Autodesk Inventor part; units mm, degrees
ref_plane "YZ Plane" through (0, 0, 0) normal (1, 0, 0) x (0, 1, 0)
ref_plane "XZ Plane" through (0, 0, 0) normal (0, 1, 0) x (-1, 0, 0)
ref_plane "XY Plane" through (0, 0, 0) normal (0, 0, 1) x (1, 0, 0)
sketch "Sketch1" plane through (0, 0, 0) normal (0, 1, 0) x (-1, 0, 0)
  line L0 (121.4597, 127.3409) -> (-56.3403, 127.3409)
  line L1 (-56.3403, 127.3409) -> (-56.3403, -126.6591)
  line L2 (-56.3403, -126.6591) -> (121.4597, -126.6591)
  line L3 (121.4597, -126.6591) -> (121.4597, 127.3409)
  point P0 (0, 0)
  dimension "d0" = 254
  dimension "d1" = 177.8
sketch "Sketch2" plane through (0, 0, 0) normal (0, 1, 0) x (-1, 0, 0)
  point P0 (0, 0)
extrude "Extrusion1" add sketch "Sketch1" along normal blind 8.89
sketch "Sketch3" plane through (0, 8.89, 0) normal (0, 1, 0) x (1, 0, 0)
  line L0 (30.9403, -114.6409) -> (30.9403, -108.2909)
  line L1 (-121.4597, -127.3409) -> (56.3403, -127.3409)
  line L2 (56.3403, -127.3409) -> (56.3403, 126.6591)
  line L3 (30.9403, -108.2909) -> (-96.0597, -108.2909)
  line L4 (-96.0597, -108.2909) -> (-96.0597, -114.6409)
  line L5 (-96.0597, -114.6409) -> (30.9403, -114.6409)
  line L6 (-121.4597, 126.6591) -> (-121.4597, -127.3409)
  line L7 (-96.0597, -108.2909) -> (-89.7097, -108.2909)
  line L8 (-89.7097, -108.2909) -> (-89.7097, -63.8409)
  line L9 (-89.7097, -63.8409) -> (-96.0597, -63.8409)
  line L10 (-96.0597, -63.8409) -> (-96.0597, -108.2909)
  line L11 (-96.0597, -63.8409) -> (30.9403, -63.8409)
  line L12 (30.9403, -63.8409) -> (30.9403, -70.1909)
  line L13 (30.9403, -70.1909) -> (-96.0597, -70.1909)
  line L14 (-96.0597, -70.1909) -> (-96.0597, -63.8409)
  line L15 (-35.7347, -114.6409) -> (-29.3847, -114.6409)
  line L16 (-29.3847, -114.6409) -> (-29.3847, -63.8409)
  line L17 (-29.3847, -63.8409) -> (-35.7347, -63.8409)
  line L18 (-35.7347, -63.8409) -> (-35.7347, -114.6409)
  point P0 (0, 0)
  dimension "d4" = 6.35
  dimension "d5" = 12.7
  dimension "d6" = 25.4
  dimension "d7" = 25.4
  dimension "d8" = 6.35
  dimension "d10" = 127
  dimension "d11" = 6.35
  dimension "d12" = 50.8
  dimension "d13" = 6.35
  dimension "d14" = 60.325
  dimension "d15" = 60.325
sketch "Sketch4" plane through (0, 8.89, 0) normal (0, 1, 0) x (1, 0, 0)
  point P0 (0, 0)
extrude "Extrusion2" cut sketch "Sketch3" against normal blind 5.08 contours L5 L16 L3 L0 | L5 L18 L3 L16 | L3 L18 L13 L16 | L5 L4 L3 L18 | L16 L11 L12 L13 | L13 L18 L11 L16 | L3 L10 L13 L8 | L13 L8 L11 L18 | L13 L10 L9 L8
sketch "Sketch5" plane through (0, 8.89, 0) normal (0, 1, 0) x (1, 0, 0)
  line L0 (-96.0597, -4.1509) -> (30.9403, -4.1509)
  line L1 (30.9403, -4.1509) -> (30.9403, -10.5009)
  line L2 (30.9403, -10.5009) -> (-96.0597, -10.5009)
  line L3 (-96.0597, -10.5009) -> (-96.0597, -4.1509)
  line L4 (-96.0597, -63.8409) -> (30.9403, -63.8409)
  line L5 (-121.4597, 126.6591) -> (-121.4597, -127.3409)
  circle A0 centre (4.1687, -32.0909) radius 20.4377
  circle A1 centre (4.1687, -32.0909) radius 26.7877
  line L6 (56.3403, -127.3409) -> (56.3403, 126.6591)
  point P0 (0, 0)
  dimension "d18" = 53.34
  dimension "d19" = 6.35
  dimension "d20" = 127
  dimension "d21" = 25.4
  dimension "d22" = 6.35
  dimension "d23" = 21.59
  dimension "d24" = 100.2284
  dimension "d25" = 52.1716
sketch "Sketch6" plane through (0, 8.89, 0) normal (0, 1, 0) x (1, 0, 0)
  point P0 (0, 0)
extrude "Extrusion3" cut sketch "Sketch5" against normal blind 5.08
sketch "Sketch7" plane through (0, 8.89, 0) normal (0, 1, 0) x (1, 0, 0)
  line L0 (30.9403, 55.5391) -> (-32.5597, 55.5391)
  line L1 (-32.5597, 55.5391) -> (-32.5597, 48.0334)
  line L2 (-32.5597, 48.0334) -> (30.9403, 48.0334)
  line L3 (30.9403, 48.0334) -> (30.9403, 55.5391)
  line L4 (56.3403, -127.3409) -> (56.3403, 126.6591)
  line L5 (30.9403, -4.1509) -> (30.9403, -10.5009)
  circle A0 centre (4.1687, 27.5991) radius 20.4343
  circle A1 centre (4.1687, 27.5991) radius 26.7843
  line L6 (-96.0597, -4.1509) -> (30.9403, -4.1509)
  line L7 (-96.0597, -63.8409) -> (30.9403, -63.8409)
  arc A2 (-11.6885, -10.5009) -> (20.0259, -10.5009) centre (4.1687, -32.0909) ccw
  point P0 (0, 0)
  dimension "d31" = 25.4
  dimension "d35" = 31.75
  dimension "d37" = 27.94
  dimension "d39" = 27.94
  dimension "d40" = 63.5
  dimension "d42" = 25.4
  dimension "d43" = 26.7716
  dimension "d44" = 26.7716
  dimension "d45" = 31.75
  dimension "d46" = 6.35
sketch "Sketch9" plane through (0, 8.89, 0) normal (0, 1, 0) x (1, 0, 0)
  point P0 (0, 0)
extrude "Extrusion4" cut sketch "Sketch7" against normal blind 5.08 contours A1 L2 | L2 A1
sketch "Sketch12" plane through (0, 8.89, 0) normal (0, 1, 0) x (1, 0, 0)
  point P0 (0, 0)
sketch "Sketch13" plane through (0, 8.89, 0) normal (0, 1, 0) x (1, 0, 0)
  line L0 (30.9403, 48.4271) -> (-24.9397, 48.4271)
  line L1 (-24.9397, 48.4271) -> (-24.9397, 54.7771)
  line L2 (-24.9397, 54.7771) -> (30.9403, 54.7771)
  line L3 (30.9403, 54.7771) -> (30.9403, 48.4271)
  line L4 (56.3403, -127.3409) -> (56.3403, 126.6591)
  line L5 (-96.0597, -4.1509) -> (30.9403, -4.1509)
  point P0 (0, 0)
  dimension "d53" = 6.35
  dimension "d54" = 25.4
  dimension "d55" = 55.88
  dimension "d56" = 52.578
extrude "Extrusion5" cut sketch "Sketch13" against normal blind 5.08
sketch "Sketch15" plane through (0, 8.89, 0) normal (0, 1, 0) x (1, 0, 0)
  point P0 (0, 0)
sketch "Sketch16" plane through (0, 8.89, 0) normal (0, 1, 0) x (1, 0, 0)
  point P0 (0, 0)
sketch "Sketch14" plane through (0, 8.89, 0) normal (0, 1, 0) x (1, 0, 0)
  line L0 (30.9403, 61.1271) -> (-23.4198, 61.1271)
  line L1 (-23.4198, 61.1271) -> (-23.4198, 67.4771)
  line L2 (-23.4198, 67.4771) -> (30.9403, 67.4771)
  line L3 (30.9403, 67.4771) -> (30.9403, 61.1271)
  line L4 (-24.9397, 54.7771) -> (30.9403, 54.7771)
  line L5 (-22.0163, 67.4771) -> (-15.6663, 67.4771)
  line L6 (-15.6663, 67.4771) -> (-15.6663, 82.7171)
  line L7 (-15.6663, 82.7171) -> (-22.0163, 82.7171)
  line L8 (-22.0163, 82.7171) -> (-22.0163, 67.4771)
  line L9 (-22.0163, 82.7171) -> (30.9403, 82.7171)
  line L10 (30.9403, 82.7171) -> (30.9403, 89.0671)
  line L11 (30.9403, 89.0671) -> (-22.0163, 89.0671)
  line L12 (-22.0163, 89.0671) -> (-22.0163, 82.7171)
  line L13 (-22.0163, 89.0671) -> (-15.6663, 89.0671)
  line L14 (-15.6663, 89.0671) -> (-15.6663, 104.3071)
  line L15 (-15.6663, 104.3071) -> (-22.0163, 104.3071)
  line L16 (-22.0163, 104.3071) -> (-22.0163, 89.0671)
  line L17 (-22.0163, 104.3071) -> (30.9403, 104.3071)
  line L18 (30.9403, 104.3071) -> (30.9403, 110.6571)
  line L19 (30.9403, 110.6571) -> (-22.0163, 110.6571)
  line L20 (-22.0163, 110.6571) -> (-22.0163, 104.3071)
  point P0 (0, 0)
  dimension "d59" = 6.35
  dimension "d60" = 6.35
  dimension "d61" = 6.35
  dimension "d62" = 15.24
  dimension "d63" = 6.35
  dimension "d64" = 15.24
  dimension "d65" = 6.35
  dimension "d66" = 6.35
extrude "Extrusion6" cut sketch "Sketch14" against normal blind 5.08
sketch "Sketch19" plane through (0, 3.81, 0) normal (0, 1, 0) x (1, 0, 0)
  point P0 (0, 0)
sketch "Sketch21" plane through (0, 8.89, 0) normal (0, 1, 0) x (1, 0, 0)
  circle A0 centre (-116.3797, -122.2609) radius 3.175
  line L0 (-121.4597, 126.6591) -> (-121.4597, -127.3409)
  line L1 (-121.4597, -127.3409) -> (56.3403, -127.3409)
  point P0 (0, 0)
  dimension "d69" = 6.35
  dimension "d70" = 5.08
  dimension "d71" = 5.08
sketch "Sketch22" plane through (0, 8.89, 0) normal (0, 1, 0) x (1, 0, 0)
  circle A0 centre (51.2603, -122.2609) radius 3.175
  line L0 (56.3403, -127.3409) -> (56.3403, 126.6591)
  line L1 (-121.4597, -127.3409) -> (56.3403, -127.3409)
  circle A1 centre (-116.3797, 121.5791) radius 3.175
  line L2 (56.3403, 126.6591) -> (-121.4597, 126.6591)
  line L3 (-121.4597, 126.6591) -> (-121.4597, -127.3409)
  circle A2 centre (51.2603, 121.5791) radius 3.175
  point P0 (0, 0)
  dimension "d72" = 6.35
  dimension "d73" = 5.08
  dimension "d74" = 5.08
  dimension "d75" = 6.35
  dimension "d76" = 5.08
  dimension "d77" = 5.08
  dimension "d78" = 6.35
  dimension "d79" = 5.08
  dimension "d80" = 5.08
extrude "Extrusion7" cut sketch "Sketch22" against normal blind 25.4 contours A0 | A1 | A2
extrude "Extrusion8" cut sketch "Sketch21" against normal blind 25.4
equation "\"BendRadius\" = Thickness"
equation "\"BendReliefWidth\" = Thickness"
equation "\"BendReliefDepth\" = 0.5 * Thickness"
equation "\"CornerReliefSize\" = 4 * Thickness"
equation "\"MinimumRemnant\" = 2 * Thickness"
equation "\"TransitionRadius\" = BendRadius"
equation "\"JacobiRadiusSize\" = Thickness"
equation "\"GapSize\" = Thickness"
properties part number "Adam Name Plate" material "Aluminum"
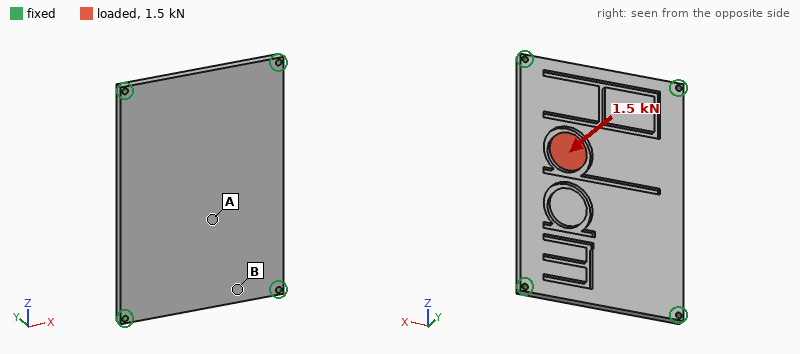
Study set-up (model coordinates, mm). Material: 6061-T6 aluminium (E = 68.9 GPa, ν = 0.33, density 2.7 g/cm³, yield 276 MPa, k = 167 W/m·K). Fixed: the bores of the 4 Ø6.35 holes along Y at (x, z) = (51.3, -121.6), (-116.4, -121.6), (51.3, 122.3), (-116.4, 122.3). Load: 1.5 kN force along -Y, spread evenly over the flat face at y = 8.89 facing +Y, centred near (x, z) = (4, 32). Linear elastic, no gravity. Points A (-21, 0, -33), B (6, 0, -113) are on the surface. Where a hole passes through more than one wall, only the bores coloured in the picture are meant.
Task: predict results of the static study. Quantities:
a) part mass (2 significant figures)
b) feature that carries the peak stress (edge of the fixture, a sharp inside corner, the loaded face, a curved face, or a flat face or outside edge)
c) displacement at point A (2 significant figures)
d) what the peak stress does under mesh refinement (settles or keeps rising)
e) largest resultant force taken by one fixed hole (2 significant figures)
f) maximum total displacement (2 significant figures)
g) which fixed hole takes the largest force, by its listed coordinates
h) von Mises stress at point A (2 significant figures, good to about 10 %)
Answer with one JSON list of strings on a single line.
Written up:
["1000 g", "edge of the fixture", "0.31 mm", "keeps rising", "1.3 kN", "0.45 mm", "(51.3, 122.3)", "13 MPa"]
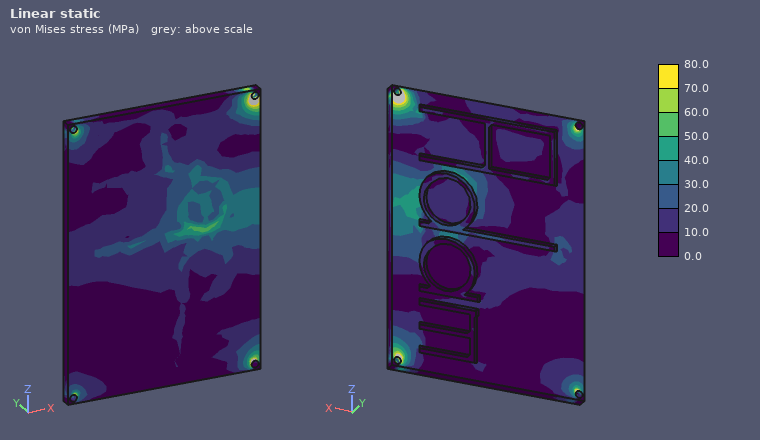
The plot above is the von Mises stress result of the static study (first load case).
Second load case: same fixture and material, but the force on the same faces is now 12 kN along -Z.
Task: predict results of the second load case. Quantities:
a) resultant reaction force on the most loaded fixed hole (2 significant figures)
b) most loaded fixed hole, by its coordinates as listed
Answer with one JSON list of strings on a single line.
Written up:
["4.6 kN", "(51.3, 122.3)"]
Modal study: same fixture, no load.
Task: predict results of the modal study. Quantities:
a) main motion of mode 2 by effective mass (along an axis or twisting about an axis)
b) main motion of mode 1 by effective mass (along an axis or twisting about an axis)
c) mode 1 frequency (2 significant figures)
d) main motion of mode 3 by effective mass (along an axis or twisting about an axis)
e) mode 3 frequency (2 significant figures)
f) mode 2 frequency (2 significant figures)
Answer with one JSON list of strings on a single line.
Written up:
["twisting about Z", "along Y", "490 Hz", "twisting about X", "1200 Hz", "900 Hz"]
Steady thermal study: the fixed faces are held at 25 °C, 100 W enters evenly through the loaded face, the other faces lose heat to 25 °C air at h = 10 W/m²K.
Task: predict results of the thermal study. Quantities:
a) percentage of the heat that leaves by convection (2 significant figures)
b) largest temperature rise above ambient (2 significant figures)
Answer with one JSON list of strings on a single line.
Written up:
["21 %", "53 K"]
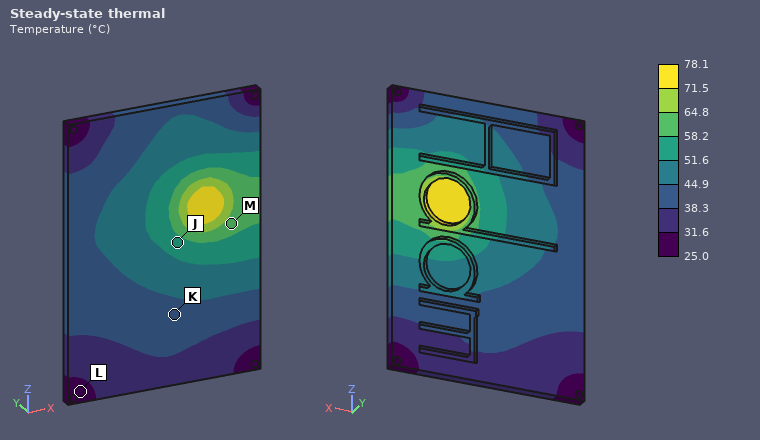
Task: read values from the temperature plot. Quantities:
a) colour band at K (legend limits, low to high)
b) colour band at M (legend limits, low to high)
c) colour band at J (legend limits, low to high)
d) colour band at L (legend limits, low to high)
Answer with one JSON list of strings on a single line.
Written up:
["38.3 to 44.9 °C", "58.2 to 64.8 °C", "51.6 to 58.2 °C", "25.0 to 31.6 °C"]
